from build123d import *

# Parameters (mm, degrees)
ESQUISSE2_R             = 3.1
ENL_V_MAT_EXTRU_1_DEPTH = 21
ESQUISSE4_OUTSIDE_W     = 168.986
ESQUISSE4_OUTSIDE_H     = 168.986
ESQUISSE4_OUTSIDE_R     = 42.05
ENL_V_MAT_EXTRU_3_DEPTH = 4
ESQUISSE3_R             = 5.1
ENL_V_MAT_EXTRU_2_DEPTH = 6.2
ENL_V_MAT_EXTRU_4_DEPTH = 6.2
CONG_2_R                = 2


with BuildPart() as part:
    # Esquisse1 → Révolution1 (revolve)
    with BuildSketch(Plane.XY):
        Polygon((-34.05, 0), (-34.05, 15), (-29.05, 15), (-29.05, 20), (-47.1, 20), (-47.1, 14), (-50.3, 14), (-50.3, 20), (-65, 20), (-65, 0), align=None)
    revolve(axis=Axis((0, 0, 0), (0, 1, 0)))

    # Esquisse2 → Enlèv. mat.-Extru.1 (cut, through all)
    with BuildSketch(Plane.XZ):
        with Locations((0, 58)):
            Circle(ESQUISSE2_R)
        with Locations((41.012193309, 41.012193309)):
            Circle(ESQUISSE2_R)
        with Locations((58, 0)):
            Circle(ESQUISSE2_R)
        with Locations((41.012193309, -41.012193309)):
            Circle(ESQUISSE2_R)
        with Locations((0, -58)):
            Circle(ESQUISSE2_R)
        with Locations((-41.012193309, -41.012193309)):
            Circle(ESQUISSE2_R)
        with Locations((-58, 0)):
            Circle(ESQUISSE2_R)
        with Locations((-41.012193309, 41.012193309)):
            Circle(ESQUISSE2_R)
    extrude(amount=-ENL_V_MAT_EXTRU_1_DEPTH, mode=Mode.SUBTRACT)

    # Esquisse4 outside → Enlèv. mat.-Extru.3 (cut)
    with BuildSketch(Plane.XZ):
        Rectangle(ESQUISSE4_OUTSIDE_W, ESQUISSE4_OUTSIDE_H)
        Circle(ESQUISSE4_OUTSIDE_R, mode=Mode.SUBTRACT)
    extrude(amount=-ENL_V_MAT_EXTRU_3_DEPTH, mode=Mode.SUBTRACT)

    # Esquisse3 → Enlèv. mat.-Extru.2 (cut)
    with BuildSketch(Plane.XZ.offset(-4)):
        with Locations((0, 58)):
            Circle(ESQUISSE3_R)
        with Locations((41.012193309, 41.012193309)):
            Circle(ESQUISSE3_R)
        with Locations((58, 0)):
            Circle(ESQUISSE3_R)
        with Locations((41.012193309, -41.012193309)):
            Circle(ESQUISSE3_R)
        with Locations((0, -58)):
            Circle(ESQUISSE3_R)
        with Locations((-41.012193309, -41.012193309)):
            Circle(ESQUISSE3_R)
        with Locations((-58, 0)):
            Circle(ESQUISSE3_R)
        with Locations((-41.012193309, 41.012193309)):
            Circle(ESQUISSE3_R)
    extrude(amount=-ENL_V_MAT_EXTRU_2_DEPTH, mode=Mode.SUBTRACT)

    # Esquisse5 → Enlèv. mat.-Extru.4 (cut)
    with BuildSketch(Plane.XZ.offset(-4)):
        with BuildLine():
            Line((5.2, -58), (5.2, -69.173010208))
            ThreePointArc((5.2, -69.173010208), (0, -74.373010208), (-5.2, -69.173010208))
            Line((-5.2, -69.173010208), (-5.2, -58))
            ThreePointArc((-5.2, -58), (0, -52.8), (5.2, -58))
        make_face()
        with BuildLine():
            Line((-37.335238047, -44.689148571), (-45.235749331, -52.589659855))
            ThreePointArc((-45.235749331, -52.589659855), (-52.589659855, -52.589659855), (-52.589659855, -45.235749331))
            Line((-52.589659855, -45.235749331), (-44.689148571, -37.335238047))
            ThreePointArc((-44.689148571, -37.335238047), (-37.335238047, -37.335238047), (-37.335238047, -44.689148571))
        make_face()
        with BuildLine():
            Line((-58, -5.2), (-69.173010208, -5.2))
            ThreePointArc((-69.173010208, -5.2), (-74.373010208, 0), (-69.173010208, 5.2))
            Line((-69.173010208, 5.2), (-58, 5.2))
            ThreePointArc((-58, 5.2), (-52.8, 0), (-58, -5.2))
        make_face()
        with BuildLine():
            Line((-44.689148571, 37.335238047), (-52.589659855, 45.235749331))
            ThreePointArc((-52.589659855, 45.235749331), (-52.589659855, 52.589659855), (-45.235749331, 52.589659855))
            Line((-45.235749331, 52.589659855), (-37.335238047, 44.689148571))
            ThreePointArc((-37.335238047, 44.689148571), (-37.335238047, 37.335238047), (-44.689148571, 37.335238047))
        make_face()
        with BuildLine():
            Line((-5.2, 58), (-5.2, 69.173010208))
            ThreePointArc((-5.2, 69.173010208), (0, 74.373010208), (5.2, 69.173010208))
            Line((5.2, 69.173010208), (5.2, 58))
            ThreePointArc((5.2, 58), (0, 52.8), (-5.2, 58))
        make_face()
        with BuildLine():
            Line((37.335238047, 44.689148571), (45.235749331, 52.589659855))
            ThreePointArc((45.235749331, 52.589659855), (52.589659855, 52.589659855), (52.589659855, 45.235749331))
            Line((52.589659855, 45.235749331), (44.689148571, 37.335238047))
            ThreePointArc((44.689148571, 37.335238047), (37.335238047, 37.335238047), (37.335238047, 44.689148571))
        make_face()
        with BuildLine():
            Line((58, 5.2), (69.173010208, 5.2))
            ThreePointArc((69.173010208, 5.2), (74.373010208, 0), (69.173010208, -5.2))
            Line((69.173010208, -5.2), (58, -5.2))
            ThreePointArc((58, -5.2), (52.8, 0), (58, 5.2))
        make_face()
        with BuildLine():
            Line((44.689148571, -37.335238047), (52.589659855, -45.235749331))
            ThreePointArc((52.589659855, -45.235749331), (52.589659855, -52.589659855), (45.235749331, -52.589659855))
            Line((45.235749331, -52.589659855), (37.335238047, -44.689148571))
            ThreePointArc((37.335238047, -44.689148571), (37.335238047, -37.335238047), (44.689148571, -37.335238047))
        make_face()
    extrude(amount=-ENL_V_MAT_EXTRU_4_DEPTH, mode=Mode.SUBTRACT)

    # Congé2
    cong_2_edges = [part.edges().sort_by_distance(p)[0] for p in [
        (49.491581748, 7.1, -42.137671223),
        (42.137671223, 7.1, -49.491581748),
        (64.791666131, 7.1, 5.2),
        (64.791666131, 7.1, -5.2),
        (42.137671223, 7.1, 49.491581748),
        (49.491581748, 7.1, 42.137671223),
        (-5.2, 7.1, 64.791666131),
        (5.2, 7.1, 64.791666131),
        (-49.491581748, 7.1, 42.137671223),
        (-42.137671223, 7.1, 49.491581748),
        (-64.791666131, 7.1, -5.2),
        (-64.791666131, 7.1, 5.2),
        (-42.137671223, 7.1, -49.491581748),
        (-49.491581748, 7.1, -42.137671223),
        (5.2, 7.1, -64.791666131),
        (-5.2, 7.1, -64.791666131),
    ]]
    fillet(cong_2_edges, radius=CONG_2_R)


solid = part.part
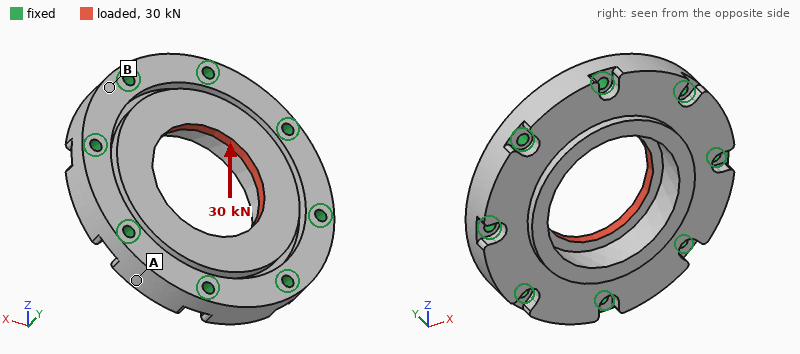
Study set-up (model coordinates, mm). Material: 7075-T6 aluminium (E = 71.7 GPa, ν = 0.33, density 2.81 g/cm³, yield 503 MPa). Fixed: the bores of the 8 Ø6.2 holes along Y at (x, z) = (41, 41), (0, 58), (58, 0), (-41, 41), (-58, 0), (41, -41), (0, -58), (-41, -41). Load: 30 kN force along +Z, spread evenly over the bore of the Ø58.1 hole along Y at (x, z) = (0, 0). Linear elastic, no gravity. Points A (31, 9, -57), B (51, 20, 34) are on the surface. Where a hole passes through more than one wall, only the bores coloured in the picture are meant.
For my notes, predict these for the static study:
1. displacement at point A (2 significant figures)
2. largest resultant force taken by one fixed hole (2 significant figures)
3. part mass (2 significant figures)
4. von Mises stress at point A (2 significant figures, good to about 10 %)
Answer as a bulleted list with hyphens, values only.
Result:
- 5.2 µm
- 4.8 kN
- 430 g
- 10 MPa
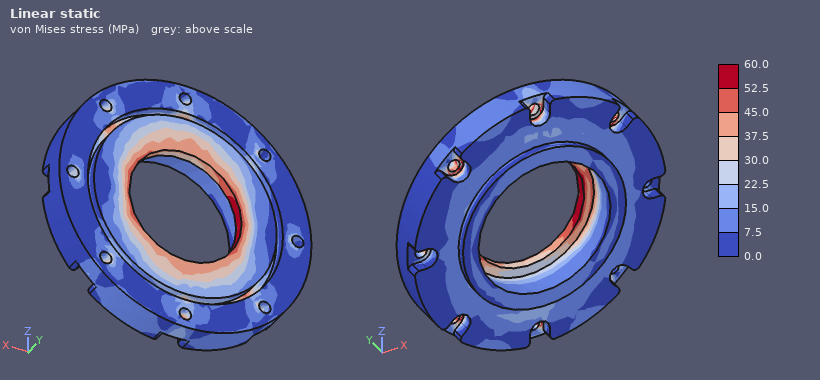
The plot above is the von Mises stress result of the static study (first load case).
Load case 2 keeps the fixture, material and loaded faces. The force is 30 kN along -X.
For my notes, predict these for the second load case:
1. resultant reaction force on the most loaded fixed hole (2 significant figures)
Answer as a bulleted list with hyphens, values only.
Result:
- 4.8 kN
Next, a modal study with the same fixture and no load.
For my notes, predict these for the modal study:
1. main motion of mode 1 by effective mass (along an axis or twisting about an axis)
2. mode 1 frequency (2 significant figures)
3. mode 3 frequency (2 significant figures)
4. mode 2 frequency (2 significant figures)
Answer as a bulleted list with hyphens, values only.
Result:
- along Y
- 9600 Hz
- 12 kHz
- 12 kHz
